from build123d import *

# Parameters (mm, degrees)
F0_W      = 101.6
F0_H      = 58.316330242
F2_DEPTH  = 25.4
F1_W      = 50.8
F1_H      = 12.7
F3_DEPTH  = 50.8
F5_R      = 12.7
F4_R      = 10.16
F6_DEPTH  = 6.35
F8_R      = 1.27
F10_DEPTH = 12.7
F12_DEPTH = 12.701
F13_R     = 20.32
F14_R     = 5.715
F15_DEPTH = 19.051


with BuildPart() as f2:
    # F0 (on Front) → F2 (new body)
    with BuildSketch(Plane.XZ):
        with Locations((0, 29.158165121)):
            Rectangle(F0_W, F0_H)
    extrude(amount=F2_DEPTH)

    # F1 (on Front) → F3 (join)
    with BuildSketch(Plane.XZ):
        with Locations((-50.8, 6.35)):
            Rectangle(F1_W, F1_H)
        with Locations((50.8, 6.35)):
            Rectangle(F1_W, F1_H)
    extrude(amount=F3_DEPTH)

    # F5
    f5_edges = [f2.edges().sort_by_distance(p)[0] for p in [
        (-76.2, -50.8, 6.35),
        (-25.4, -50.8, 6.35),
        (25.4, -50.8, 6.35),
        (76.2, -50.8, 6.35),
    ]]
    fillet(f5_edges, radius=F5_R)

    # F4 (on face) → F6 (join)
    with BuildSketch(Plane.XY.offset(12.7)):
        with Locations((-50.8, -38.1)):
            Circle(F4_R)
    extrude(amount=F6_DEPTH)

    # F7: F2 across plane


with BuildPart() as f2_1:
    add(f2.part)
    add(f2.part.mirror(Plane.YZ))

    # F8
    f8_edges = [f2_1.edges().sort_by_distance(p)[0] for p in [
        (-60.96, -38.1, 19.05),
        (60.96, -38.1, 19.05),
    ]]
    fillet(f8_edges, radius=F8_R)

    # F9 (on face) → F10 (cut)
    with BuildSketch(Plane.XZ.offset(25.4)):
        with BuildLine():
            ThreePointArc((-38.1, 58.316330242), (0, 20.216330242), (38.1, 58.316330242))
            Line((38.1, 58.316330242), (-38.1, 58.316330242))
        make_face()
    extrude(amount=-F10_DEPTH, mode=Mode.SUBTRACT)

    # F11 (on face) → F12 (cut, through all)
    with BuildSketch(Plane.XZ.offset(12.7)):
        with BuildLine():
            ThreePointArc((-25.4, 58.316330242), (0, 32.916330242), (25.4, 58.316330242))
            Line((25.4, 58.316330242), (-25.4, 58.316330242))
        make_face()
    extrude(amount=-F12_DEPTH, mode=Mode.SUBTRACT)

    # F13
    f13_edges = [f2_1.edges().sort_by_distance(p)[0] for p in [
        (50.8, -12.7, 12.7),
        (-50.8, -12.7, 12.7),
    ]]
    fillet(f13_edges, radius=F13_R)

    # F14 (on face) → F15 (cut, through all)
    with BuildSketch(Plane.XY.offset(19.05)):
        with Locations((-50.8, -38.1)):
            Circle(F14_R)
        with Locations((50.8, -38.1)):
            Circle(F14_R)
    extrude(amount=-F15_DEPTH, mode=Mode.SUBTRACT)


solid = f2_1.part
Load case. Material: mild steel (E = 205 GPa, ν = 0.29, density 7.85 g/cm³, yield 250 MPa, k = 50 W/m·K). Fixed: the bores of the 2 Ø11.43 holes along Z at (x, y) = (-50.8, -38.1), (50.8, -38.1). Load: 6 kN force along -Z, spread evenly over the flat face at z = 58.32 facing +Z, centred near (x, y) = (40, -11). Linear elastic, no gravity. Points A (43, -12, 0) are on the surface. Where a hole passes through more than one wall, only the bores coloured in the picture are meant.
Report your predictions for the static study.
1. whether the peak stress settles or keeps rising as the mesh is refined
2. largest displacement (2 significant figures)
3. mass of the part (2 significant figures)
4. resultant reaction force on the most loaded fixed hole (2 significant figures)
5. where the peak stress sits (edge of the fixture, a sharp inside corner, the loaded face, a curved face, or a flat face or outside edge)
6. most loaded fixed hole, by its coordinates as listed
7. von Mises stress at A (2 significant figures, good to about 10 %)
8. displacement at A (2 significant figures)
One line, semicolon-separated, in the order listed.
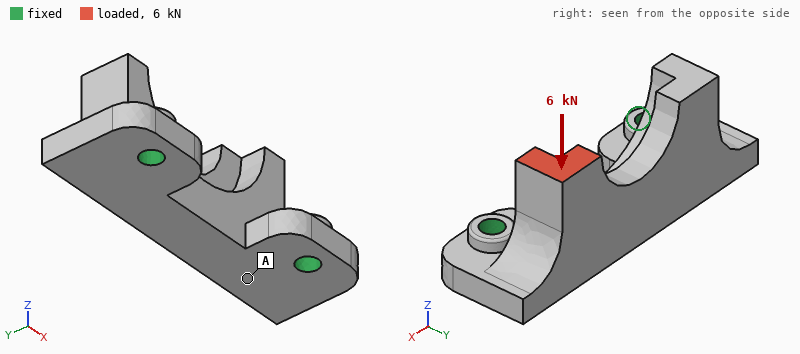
keeps rising; 46 µm; 1.3 kg; 5.3 kN; edge of the fixture; (50.8, -38.1); 9.8 MPa; 15 µm
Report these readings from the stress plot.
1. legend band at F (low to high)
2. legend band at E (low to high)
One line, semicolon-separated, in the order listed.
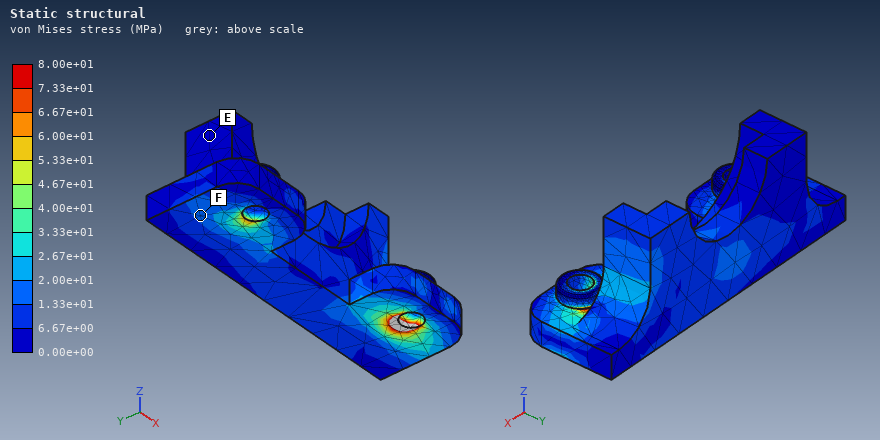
1.33e+01 to 2.00e+01 MPa; 0.00e+00 to 6.67e+00 MPa
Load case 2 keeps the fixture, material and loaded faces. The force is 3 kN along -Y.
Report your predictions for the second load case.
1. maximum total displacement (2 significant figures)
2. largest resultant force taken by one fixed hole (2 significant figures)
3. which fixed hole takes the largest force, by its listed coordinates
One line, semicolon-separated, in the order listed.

79 µm; 2.8 kN; (50.8, -38.1)
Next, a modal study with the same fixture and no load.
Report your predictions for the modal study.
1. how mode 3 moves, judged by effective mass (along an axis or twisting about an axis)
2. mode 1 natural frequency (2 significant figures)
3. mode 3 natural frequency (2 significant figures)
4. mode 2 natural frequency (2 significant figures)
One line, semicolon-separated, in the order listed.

along Z; 2400 Hz; 6500 Hz; 4400 Hz
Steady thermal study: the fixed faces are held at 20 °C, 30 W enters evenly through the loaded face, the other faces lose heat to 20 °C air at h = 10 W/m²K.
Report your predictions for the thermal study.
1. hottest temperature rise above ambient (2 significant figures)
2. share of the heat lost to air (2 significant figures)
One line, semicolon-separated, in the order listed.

55 K; 10 %
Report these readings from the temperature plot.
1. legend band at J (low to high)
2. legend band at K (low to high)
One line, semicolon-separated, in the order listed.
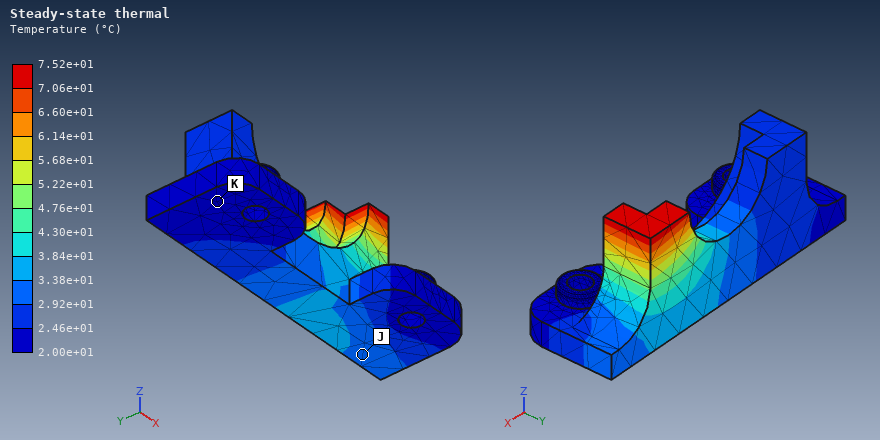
2.92e+01 to 3.38e+01 °C; 2.00e+01 to 2.46e+01 °C
